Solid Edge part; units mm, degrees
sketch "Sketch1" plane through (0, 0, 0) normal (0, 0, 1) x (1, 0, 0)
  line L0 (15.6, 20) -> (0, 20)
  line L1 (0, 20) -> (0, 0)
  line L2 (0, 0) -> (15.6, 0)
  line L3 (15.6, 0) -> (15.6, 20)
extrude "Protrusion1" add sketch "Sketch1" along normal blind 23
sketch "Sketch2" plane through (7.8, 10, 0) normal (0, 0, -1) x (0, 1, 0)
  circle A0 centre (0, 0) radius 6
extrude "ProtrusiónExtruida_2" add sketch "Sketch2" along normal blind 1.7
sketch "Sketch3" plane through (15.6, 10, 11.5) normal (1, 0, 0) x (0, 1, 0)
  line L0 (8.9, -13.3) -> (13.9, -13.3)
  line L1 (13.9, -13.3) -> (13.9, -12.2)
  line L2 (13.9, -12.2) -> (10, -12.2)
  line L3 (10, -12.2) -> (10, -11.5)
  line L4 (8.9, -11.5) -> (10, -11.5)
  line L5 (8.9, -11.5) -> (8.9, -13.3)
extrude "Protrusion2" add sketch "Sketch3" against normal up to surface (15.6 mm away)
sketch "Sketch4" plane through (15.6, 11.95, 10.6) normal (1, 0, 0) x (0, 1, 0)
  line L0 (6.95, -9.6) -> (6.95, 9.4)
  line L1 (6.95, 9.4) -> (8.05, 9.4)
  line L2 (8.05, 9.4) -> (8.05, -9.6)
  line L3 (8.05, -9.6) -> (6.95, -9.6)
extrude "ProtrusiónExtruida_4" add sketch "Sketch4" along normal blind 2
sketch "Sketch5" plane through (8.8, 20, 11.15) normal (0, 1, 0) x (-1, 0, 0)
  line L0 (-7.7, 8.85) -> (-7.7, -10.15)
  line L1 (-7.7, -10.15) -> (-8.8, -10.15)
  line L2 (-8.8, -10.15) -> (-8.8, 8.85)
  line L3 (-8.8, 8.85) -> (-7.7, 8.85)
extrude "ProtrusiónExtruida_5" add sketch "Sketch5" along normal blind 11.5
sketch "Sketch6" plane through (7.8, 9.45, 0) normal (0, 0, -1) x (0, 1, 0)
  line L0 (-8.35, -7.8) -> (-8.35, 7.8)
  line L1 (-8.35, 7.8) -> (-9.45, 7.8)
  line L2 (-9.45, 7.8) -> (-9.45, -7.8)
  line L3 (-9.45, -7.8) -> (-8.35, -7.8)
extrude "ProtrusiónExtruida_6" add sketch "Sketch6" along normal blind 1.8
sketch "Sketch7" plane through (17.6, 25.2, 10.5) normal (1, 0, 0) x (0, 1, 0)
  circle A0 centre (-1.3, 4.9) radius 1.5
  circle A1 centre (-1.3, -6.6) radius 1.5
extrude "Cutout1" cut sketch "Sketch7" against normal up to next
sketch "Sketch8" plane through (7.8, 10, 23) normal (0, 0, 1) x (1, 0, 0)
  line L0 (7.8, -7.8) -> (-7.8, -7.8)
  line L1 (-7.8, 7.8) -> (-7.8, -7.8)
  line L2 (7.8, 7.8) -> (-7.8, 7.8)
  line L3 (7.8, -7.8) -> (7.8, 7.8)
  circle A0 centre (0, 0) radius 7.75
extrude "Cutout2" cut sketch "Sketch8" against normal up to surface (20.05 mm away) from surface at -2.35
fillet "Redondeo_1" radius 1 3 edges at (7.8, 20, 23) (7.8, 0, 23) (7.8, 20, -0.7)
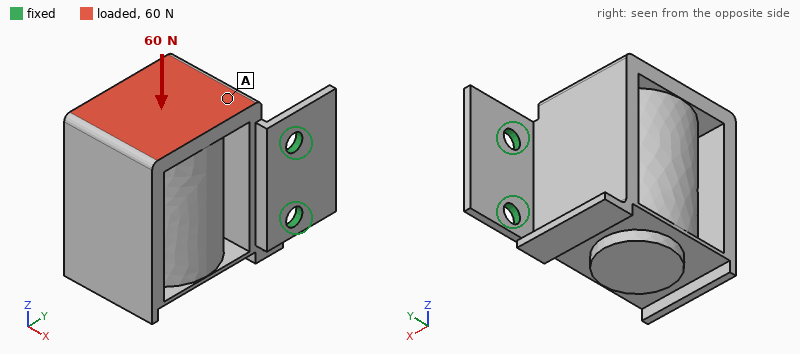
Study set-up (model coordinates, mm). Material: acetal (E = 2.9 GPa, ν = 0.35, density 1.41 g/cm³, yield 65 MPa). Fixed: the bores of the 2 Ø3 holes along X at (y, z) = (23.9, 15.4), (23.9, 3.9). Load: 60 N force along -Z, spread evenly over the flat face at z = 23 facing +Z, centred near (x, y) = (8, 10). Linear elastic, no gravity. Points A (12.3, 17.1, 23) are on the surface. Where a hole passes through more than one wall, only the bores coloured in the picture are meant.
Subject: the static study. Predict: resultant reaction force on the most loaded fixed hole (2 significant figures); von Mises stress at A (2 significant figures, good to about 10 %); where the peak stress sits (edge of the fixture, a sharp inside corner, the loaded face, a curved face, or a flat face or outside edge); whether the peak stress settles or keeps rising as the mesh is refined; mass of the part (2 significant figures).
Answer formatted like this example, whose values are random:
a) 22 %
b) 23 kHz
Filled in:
a) 81 N
b) 4.6 MPa
c) edge of the fixture
d) keeps rising
e) 9.4 g
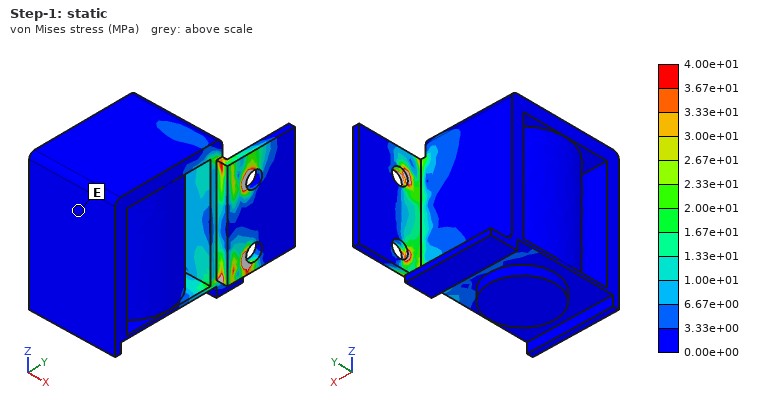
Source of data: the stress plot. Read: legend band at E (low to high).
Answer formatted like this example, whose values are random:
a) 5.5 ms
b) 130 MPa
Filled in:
a) 0.00e+00 to 3.33e+00 MPa
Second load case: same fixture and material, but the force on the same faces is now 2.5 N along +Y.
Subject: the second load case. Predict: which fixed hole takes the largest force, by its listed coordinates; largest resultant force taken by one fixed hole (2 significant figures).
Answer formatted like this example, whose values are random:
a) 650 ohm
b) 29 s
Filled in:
a) (23.9, 15.4)
b) 3.8 N
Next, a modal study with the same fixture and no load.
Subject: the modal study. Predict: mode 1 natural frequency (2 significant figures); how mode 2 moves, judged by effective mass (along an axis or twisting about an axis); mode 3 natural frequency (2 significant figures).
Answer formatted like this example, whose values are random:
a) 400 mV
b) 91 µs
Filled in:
a) 120 Hz
b) along Z
c) 830 Hz
